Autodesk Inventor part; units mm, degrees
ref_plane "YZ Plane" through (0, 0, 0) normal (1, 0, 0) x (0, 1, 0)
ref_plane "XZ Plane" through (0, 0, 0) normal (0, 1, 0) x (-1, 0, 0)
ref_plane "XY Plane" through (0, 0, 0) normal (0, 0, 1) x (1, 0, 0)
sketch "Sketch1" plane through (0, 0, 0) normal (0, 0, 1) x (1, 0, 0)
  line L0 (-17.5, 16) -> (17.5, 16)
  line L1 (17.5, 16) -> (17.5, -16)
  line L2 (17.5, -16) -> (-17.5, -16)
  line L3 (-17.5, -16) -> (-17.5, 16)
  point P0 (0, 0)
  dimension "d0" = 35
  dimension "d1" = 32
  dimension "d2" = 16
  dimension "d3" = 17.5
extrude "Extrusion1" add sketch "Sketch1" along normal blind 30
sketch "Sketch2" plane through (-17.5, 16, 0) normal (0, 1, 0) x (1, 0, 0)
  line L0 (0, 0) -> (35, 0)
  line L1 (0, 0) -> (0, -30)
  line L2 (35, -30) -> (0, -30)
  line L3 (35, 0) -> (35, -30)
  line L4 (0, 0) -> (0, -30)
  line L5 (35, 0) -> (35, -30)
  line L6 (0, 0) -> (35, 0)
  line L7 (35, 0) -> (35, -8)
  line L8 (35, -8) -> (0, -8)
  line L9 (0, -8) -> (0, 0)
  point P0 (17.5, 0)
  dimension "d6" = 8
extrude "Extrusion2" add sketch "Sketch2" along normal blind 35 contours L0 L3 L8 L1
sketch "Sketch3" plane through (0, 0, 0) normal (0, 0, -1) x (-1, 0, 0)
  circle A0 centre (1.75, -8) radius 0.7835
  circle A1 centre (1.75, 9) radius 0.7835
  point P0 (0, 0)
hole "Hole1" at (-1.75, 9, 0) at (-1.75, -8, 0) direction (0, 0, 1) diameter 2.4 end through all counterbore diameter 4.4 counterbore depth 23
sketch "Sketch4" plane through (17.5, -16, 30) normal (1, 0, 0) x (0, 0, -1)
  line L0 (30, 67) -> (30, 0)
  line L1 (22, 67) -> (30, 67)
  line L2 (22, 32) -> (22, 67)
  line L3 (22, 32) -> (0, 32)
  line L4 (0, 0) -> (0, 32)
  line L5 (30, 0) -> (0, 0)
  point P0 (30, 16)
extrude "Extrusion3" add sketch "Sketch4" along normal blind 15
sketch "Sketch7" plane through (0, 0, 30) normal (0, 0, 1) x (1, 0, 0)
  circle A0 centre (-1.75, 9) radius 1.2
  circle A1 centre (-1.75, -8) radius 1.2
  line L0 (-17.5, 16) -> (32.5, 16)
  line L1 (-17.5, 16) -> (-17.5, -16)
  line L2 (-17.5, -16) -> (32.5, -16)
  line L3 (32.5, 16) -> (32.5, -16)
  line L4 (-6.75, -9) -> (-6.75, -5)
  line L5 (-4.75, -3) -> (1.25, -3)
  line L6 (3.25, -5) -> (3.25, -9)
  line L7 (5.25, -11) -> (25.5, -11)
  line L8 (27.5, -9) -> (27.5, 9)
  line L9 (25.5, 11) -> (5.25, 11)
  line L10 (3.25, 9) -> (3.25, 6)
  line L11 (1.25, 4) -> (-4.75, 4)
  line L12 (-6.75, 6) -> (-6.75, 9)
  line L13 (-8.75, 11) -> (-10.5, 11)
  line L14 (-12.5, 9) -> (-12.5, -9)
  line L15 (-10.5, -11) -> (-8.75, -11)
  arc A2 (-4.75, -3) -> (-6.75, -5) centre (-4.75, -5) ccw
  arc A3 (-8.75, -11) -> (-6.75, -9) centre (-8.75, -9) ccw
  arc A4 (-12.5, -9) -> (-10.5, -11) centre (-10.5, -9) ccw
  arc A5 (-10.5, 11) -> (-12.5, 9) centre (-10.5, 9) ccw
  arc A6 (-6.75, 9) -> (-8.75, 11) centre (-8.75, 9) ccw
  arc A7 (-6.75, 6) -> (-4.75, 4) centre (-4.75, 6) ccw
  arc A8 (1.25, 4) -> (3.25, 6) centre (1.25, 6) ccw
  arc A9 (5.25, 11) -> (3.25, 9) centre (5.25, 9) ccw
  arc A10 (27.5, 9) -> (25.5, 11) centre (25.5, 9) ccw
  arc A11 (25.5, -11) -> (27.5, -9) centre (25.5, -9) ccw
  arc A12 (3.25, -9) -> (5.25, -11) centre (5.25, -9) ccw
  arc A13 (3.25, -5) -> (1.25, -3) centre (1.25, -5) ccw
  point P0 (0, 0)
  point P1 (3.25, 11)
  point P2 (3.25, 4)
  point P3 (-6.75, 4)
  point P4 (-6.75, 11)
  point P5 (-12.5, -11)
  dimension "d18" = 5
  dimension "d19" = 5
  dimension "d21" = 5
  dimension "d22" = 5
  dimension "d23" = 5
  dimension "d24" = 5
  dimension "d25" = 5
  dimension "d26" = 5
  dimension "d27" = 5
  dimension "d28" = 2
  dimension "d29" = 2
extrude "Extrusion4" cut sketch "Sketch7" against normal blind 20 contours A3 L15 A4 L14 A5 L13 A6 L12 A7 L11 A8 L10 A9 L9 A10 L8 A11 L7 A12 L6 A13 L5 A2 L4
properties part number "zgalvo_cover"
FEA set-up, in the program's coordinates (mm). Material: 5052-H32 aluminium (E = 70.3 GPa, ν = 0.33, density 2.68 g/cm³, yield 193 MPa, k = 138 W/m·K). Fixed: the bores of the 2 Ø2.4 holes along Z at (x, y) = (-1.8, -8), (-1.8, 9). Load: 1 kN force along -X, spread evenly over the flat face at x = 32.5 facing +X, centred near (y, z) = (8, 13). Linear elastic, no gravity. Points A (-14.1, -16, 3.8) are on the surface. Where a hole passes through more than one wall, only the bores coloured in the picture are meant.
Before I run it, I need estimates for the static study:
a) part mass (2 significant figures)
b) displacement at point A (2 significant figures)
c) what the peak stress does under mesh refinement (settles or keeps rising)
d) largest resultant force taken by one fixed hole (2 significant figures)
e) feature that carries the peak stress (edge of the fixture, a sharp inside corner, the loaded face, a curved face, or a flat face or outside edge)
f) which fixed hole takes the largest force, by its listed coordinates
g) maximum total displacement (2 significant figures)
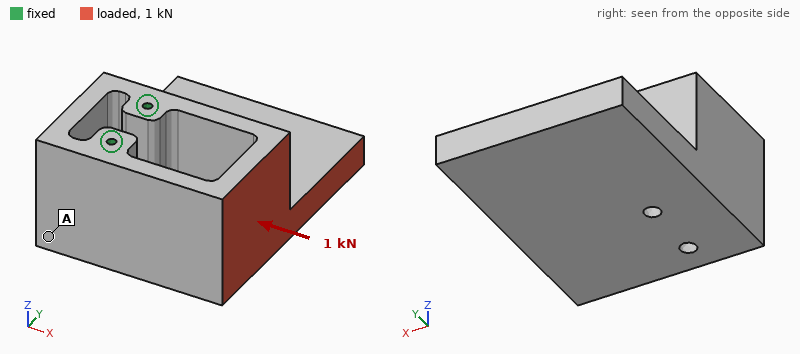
130 g
26 µm
keeps rising
780 N
edge of the fixture
(-1.8, 9)
66 µm
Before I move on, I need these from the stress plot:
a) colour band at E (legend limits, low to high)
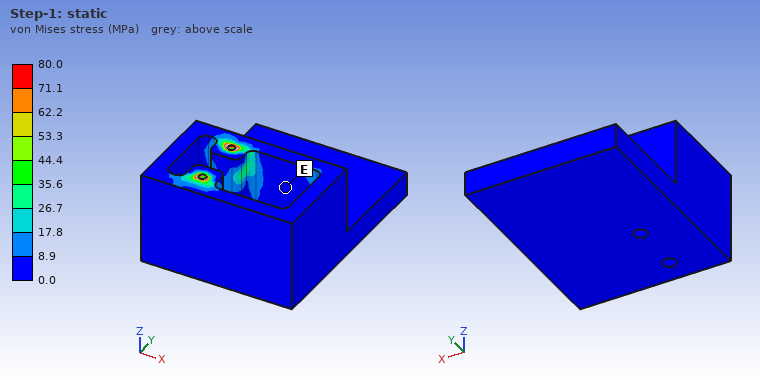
0.0 to 8.9 MPa
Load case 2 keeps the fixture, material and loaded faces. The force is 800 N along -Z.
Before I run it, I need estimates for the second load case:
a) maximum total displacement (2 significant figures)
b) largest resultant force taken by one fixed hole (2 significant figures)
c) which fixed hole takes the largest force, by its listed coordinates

0.13 mm
660 N
(-1.8, 9)
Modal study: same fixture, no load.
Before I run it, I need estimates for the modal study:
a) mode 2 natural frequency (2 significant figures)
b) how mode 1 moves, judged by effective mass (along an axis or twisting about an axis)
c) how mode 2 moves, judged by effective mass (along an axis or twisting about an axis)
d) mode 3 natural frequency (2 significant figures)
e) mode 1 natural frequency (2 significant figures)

2600 Hz
along X
along Y
3200 Hz
1800 Hz
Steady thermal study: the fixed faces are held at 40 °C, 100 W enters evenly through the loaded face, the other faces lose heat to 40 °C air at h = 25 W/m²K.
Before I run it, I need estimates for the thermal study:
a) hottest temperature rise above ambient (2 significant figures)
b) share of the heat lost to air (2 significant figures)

66 K
13 %
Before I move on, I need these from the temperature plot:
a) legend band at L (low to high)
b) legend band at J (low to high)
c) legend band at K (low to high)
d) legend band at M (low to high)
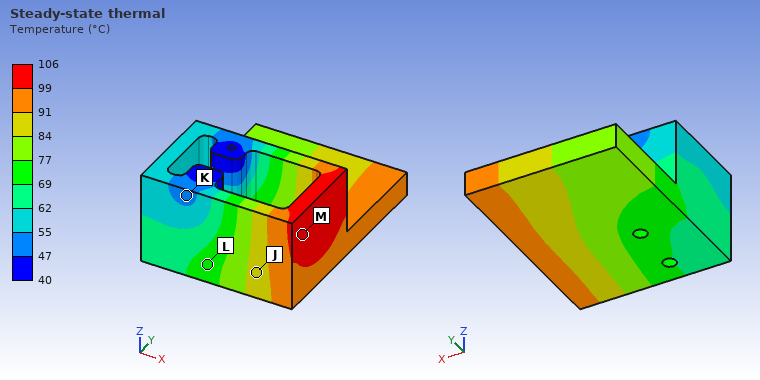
69 to 77 °C
84 to 91 °C
47 to 55 °C
99 to 106 °C
